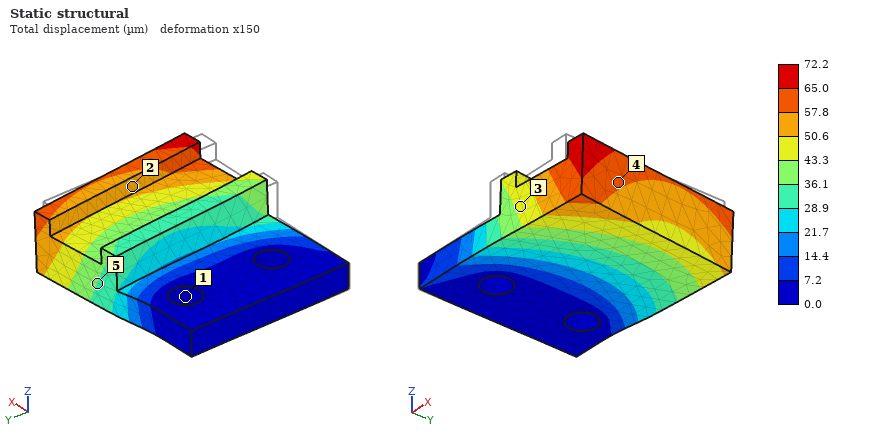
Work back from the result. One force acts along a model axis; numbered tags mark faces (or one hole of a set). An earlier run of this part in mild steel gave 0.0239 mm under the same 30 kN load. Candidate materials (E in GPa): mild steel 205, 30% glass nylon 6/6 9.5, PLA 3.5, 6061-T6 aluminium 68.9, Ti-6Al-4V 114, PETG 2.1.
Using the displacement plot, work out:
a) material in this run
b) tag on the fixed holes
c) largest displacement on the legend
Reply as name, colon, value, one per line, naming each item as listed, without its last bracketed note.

material in this run: 6061-T6 aluminium
tag on the fixed holes: 1
largest displacement on the legend: 72.2 µm
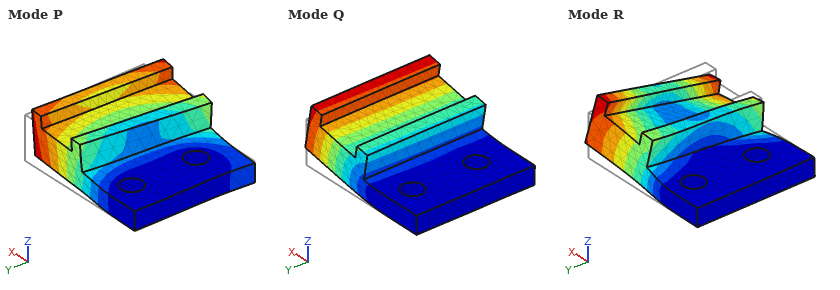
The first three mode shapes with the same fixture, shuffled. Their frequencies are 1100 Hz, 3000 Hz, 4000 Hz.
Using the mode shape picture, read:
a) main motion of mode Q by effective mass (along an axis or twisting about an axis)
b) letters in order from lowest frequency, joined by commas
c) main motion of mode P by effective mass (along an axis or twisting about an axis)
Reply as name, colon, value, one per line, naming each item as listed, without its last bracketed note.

main motion of mode Q by effective mass: along Z
letters in order from lowest frequency, joined by commas: Q, R, P
main motion of mode P by effective mass: along Y
